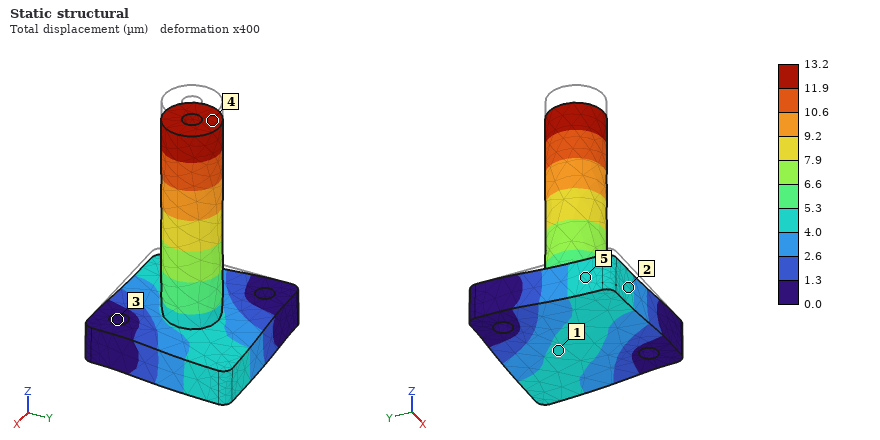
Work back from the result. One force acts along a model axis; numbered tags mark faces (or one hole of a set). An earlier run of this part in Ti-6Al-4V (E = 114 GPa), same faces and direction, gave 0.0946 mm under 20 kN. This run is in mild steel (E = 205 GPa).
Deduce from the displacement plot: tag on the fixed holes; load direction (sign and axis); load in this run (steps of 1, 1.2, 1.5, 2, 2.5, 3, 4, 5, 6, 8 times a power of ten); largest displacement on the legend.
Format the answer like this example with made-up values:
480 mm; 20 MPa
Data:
3; -Z; 5 kN; 13.2 µm
